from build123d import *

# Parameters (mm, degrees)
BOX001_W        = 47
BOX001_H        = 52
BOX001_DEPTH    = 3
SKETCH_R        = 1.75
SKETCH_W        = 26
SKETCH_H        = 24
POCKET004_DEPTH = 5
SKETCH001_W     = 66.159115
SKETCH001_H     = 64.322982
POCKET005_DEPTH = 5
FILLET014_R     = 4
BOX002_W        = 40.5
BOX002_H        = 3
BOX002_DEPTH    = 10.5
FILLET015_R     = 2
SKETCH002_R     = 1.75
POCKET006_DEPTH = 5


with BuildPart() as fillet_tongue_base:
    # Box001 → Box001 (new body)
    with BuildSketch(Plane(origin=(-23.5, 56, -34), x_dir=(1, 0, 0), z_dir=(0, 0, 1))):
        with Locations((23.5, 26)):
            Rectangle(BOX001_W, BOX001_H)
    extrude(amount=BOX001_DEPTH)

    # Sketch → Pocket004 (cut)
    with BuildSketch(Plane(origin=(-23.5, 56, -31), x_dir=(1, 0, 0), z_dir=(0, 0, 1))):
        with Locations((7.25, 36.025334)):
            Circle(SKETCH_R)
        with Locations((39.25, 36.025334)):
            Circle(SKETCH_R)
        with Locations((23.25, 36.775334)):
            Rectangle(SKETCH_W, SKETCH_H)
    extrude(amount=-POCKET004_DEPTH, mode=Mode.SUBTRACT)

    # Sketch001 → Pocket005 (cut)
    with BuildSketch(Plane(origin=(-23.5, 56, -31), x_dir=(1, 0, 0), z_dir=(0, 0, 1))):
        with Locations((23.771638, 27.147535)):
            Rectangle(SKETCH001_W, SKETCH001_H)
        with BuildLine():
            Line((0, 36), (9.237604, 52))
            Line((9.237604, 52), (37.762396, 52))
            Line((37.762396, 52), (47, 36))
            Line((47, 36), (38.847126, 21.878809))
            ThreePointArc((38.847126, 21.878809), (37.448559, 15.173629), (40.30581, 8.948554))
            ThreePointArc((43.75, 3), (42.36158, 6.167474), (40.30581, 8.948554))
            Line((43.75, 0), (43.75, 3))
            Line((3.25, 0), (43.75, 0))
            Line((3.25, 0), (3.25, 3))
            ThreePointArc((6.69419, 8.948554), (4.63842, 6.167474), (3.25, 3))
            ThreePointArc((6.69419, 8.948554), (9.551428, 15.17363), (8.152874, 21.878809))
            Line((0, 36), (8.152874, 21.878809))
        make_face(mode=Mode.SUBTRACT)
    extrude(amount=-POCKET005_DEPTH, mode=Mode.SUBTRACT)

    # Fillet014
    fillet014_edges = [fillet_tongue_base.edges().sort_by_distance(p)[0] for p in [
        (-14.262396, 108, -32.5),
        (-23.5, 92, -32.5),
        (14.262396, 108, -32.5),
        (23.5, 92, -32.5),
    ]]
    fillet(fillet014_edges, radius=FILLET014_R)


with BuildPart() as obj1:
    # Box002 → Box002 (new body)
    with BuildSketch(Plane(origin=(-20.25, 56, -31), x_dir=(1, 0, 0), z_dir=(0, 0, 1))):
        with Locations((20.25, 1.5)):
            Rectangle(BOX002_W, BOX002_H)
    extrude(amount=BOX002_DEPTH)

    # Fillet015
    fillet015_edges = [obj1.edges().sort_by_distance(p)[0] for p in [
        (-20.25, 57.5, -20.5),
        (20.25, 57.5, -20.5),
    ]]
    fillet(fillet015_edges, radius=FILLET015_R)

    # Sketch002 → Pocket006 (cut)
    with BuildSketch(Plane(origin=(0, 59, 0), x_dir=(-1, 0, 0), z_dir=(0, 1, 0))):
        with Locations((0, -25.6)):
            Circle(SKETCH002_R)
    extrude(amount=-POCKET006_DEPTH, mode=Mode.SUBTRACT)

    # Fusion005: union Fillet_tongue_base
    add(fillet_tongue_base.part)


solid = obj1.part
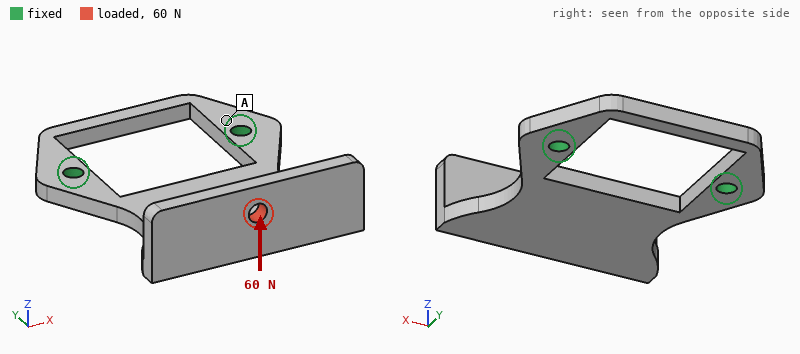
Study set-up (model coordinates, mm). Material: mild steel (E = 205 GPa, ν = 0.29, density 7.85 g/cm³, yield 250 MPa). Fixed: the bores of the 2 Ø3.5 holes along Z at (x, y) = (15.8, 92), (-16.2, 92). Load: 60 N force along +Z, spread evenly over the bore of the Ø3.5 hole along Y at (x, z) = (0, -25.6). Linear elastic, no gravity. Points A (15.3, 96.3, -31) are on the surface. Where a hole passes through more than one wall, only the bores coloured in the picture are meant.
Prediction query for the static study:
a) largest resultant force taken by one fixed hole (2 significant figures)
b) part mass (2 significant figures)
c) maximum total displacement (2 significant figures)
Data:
30 N
39 g
0.16 mm
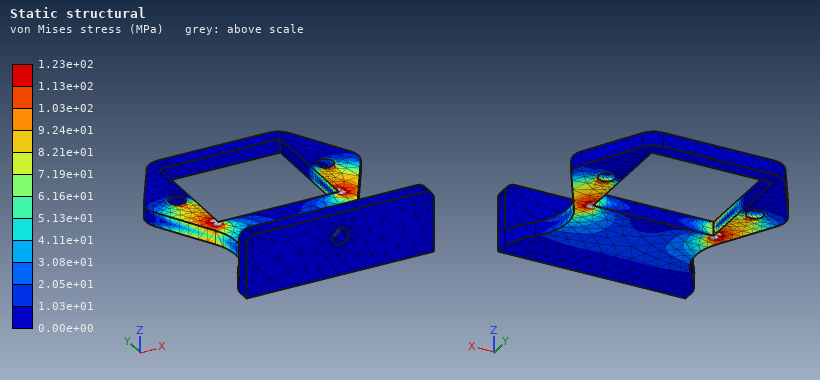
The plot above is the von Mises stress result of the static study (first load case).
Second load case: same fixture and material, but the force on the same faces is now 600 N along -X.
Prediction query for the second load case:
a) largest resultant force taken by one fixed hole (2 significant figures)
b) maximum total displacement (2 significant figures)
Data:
600 N
0.12 mm
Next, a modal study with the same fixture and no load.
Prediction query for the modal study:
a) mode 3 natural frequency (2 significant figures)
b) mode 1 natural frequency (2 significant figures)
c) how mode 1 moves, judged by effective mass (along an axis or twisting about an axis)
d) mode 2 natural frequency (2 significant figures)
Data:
5600 Hz
760 Hz
along Z
2600 Hz
